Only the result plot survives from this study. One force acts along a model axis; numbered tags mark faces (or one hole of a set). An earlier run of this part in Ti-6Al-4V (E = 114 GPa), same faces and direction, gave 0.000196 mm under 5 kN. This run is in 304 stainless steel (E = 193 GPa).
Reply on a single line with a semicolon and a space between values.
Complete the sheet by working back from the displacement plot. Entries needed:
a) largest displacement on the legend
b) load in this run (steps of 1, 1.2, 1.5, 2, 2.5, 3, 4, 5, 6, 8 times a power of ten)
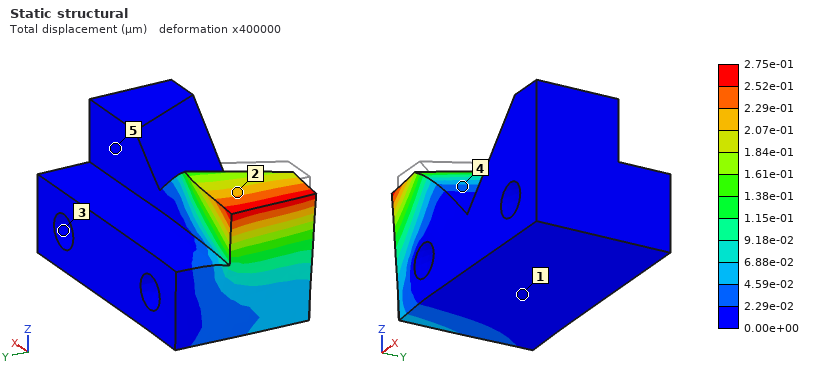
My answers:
2.75e-01 µm; 12 kN
